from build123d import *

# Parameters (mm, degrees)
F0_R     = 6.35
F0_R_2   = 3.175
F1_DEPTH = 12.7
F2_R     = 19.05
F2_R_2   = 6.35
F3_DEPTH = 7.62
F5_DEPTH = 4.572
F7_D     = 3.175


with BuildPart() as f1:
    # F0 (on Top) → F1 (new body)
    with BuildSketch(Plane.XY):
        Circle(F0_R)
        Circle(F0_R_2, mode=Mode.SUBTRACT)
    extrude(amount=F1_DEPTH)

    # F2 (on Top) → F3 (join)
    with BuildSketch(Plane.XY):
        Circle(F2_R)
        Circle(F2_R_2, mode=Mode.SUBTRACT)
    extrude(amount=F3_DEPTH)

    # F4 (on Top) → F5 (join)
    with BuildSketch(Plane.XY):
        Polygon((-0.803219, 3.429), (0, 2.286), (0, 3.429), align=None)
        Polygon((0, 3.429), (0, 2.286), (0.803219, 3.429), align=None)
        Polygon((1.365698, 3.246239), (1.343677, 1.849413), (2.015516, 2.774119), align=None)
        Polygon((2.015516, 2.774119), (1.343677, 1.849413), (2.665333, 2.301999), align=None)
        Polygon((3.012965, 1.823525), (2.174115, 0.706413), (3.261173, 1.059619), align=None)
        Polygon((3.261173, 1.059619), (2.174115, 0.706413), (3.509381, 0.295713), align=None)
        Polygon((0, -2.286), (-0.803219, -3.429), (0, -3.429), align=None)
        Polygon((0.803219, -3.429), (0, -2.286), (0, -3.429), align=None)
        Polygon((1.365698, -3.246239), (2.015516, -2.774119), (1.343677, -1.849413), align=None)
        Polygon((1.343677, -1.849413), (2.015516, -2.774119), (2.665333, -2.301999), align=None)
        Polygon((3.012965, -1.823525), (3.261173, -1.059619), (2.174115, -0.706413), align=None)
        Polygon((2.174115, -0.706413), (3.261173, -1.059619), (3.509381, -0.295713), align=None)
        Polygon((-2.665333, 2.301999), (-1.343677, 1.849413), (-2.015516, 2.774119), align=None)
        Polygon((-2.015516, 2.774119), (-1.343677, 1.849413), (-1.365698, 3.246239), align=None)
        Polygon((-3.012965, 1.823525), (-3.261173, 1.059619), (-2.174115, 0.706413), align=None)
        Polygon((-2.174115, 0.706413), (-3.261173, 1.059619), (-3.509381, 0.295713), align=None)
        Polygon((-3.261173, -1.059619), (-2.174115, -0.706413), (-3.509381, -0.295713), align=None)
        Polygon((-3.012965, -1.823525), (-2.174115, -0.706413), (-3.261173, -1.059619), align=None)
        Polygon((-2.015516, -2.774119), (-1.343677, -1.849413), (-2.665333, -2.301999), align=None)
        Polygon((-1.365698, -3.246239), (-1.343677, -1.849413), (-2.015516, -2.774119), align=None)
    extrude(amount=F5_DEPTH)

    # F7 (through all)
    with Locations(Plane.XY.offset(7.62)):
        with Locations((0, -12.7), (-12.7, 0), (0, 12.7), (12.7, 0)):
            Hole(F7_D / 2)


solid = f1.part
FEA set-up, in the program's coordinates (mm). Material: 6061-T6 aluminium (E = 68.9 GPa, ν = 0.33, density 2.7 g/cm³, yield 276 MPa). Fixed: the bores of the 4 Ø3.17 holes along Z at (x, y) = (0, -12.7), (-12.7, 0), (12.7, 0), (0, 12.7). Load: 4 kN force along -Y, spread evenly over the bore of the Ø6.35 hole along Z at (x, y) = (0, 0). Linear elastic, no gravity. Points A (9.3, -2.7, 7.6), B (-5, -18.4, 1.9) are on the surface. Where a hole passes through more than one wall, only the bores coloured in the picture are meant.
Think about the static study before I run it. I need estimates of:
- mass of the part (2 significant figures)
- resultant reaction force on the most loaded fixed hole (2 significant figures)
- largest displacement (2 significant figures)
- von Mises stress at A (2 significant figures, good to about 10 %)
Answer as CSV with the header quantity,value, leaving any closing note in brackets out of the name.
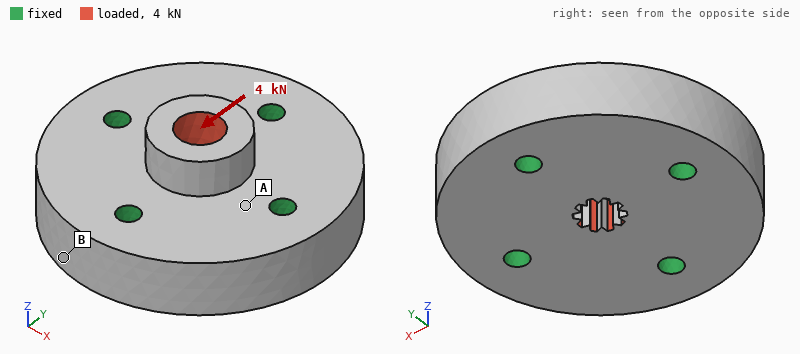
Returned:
quantity,value
mass of the part,24 g
resultant reaction force on the most loaded fixed hole,1.4 kN
largest displacement,11 µm
von Mises stress at A,11 MPa
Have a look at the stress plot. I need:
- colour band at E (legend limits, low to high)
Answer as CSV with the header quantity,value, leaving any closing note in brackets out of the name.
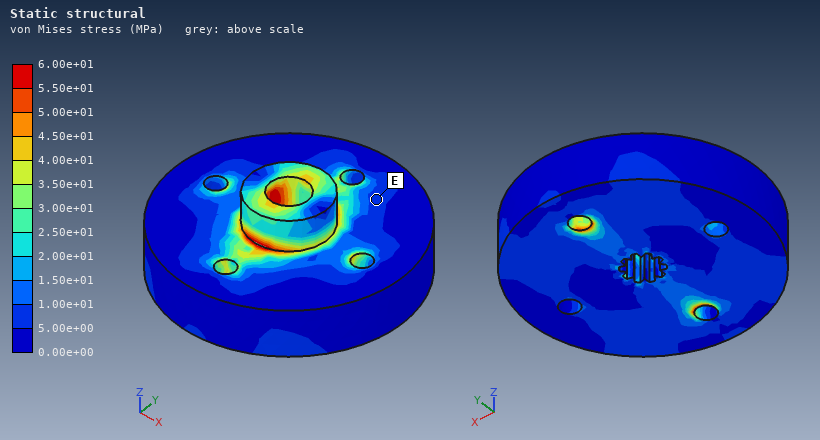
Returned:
quantity,value
colour band at E,5.00e+00 to 1.00e+01 MPa
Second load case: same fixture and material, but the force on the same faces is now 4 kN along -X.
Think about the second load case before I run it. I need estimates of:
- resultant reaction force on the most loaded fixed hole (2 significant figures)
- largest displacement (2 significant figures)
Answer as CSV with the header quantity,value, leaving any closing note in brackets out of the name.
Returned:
quantity,value
resultant reaction force on the most loaded fixed hole,1.4 kN
largest displacement,11 µm
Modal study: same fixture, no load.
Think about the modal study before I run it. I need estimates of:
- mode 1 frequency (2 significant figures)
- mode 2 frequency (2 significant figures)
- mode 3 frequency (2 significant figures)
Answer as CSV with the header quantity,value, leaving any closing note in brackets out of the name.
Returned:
quantity,value
mode 1 frequency,43 kHz
mode 2 frequency,45 kHz
mode 3 frequency,45 kHz
